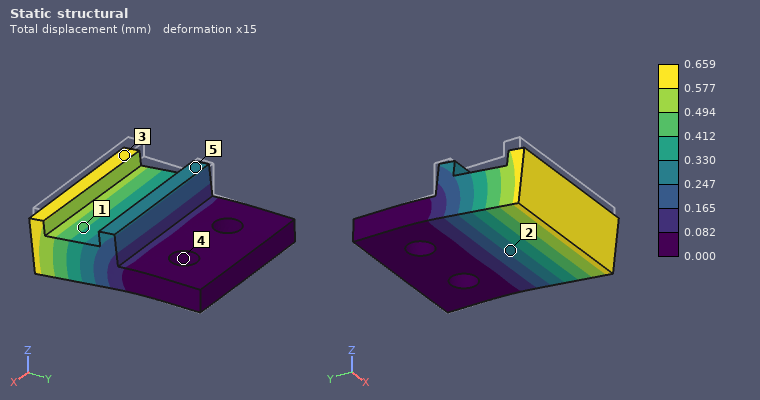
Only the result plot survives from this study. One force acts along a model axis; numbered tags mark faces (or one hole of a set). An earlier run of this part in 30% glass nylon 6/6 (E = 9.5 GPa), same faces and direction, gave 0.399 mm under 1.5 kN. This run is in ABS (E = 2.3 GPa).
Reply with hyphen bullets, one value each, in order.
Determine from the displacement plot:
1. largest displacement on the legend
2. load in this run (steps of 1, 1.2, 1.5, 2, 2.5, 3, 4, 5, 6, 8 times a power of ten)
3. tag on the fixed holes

- 0.659 mm
- 600 N
- 4
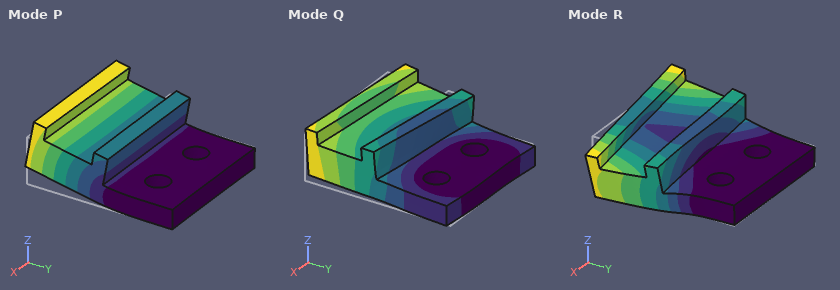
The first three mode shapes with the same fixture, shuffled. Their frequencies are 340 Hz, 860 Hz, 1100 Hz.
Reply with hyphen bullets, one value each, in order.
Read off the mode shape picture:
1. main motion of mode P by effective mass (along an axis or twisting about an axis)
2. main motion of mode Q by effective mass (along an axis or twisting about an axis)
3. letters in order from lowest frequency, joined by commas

- along Z
- along X
- P, R, Q
